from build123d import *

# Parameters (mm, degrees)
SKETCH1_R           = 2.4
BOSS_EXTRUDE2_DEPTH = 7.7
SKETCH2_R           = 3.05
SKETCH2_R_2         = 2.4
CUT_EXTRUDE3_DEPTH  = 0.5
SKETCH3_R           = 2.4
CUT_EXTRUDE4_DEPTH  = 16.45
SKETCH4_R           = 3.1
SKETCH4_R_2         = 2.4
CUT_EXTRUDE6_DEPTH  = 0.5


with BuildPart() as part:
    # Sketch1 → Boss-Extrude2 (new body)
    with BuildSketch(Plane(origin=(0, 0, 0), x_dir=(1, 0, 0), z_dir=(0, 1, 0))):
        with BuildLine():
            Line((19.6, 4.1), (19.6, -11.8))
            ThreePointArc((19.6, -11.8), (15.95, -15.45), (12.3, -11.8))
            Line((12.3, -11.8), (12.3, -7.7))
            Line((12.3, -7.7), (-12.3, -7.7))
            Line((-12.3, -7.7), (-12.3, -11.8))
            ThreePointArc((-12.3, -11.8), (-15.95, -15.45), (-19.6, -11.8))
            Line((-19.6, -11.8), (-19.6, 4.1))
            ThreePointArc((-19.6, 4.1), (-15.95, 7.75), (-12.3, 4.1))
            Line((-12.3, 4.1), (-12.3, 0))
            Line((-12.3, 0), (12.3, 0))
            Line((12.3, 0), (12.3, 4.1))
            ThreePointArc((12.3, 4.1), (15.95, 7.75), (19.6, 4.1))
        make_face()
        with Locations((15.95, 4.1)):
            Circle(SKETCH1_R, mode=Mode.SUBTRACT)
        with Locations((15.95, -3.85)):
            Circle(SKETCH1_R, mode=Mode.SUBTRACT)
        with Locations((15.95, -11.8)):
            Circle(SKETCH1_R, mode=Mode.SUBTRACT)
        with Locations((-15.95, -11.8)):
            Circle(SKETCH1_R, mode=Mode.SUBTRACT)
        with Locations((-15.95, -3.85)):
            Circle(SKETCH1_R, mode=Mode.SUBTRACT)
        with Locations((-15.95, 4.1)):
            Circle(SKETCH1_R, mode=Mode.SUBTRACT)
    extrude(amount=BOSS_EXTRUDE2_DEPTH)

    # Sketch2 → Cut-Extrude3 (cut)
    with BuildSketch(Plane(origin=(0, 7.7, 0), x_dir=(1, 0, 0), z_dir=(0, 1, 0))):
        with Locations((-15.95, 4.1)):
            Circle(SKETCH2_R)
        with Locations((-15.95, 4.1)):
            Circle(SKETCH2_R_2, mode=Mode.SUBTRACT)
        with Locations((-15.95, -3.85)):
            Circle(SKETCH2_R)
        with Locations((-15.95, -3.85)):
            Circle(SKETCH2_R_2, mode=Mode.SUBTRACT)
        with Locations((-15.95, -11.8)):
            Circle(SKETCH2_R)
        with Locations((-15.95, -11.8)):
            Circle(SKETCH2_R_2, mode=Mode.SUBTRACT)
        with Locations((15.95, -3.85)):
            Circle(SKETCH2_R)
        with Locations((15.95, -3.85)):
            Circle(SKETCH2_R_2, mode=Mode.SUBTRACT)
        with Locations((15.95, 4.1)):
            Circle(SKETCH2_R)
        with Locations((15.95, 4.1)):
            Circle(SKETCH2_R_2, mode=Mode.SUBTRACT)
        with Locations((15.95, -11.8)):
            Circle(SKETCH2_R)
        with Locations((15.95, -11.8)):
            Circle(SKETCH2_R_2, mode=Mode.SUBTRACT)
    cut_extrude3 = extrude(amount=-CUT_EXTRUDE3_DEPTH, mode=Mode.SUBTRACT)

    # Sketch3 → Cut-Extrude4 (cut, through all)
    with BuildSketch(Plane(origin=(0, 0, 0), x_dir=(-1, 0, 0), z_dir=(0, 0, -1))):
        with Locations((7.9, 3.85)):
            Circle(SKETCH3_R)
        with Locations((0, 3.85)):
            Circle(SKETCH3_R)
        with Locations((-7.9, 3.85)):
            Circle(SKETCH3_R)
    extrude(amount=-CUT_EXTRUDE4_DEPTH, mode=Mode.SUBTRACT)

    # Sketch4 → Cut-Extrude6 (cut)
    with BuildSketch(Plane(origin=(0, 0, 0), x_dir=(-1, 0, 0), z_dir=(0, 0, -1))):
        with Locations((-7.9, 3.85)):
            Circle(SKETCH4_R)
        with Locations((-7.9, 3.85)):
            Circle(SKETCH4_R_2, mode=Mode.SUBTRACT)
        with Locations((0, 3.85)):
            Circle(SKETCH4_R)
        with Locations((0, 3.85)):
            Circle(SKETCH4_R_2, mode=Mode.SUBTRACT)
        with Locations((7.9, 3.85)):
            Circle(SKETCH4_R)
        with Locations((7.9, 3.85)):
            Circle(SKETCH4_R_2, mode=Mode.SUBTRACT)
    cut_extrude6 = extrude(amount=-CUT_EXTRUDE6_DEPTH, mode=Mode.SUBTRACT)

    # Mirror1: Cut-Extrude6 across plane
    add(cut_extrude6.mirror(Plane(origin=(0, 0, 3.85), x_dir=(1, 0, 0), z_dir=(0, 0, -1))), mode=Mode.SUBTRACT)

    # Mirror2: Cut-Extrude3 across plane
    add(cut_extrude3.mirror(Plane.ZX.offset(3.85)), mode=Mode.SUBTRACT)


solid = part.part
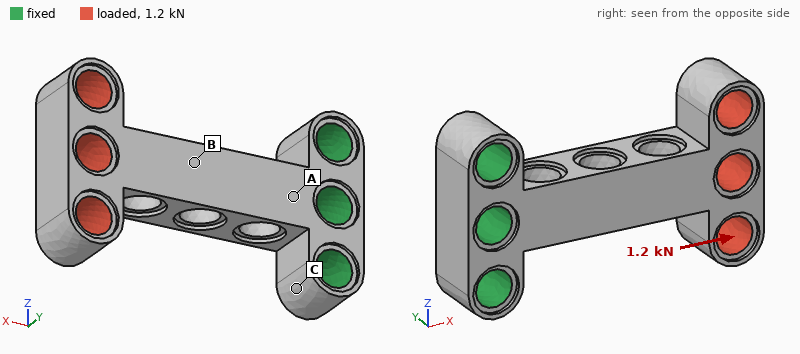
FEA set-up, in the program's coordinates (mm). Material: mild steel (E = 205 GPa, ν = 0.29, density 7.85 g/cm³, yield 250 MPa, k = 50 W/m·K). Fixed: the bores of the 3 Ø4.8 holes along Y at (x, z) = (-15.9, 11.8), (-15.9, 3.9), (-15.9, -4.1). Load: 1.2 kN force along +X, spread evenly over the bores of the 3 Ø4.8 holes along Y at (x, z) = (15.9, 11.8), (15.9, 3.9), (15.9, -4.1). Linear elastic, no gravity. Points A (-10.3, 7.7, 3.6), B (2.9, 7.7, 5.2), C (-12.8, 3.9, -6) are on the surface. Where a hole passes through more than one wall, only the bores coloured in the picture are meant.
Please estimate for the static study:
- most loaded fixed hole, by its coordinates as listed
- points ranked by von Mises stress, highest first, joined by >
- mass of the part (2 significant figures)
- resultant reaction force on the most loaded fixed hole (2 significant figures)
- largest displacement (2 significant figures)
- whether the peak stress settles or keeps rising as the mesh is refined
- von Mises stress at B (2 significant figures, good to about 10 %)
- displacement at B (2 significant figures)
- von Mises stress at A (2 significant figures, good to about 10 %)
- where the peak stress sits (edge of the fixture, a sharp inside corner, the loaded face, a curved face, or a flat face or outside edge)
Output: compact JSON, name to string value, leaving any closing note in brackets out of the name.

{"most loaded fixed hole, by its coordinates as listed": "(-15.9, 3.9)", "points ranked by von Mises stress, highest first, joined by >": "B > A > C", "mass of the part": "20 g", "resultant reaction force on the most loaded fixed hole": "970 N", "largest displacement": "11 µm", "whether the peak stress settles or keeps rising as the mesh is refined": "keeps rising", "von Mises stress at B": "57 MPa", "displacement at B": "3.6 µm", "von Mises stress at A": "45 MPa", "where the peak stress sits": "a sharp inside corner"}
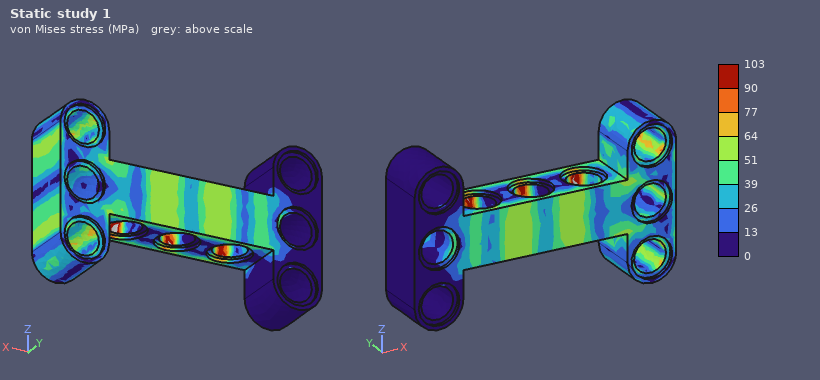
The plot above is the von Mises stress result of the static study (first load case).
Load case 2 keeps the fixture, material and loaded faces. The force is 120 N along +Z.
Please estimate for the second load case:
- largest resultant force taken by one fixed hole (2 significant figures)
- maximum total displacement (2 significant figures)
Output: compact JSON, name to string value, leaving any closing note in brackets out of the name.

{"largest resultant force taken by one fixed hole": "250 N", "maximum total displacement": "52 µm"}
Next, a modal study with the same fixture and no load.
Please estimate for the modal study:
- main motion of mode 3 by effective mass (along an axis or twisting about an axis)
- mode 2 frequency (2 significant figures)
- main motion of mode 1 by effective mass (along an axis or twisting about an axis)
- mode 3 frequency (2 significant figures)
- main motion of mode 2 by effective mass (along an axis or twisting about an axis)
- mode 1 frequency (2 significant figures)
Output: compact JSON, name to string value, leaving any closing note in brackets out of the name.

{"main motion of mode 3 by effective mass": "twisting about X", "mode 2 frequency": "3900 Hz", "main motion of mode 1 by effective mass": "along Z", "mode 3 frequency": "7400 Hz", "main motion of mode 2 by effective mass": "along Y", "mode 1 frequency": "3100 Hz"}
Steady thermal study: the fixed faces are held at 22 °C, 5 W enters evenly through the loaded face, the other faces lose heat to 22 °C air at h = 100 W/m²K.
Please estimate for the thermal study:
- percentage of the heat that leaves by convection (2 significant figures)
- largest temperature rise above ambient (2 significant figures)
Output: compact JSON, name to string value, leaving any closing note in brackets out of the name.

{"percentage of the heat that leaves by convection": "72 %", "largest temperature rise above ambient": "37 K"}
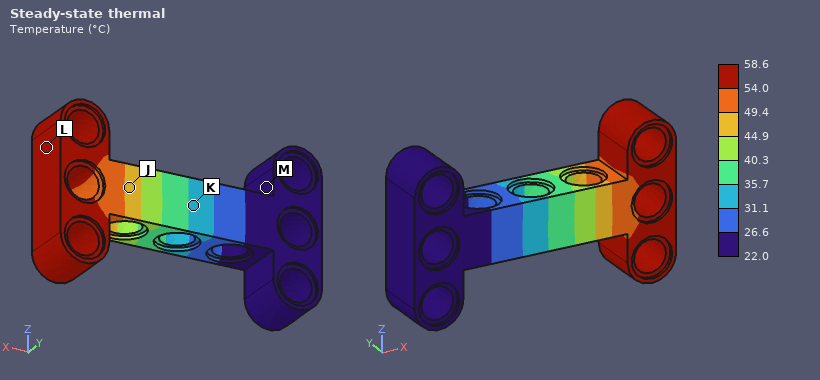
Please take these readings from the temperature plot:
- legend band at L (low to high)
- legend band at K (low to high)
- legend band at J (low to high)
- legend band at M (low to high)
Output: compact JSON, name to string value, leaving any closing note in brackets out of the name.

{"legend band at L": "54.0 to 58.6 °C", "legend band at K": "31.1 to 35.7 °C", "legend band at J": "44.9 to 49.4 °C", "legend band at M": "22.0 to 26.6 °C"}
